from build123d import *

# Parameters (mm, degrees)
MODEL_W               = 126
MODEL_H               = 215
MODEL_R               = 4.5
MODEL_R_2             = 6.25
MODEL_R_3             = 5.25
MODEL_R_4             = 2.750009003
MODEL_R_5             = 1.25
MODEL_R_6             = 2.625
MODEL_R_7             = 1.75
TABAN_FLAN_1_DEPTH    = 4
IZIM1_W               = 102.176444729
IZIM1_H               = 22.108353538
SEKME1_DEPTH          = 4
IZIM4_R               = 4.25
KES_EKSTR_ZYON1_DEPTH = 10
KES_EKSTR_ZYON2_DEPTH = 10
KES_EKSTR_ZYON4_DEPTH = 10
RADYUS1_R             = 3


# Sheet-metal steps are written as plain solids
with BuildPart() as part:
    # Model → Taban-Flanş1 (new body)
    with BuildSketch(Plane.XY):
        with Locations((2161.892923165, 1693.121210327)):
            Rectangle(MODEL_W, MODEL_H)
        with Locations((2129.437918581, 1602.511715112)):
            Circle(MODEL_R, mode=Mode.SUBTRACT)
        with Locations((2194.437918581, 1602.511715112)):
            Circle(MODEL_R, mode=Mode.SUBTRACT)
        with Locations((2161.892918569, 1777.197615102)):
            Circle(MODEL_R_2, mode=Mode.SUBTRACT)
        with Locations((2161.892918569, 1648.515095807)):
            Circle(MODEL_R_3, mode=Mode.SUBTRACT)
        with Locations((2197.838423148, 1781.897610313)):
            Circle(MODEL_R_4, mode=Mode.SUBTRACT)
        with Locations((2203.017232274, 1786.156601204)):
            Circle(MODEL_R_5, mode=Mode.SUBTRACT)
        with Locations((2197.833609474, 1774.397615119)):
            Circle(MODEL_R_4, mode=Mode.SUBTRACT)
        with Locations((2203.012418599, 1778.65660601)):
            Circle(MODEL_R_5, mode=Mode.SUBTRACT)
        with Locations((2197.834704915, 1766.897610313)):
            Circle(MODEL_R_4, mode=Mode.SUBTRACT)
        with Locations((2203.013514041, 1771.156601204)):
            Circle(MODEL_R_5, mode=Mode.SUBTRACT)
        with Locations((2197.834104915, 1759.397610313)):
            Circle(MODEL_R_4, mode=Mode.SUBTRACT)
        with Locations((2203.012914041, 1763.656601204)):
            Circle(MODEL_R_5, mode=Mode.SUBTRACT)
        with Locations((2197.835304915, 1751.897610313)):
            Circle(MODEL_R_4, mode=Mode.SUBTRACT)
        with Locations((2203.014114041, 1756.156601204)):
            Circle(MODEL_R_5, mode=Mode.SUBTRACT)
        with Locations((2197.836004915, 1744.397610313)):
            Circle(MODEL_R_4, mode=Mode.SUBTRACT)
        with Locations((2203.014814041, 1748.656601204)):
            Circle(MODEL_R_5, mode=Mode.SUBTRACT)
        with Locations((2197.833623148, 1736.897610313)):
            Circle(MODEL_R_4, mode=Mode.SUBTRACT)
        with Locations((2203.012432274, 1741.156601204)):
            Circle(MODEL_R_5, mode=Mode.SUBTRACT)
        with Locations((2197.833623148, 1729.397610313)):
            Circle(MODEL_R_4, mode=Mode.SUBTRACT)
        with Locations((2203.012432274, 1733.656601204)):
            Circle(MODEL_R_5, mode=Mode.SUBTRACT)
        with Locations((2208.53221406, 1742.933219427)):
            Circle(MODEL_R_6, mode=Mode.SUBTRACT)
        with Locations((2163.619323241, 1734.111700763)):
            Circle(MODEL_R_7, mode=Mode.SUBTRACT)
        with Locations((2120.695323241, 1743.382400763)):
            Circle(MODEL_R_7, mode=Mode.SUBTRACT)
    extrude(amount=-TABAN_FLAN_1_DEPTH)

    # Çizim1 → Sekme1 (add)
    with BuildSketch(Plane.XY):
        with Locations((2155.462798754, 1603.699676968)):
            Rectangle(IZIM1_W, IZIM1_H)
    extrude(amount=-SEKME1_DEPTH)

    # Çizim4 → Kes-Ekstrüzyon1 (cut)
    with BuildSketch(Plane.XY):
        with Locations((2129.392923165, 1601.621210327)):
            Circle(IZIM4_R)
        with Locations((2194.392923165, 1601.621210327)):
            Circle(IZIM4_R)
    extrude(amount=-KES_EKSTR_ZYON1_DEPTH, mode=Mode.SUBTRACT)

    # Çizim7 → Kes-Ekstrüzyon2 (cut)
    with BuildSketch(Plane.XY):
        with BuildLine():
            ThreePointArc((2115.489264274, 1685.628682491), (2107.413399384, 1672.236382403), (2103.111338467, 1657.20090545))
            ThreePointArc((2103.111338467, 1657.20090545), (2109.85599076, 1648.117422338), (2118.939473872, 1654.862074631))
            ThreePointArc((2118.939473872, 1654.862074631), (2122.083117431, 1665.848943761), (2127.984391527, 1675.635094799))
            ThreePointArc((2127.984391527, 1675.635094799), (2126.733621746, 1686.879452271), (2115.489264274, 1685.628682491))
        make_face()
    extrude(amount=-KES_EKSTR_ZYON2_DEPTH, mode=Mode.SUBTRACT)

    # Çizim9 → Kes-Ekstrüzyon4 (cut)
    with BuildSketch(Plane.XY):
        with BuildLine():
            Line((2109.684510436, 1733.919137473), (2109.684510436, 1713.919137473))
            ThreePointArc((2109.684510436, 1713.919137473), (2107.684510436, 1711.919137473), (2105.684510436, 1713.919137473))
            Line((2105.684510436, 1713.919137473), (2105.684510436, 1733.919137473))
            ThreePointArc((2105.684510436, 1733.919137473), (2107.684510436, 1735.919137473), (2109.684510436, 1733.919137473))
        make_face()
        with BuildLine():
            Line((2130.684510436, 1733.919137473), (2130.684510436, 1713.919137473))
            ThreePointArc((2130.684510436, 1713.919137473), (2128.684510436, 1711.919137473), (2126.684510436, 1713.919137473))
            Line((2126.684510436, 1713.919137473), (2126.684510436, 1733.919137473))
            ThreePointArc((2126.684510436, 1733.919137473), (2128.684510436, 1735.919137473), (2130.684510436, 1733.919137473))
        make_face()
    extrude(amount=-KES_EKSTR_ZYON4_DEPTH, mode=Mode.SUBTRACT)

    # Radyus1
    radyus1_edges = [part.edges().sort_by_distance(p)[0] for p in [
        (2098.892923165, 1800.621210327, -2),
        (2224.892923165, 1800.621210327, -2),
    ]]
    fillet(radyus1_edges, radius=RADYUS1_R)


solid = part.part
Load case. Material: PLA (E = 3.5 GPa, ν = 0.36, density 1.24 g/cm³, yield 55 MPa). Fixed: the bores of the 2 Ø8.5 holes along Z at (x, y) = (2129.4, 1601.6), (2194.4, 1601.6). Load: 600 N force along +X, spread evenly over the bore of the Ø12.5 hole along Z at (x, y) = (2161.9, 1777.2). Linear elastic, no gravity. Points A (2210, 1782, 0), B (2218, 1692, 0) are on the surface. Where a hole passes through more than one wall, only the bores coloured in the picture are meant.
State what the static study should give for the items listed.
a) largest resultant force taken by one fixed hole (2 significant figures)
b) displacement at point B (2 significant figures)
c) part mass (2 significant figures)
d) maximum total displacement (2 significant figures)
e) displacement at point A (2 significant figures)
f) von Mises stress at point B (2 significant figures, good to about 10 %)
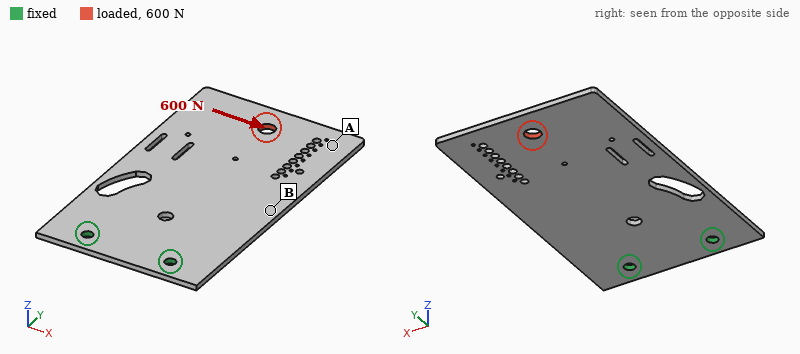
1.5 kN
0.55 mm
130 g
1.3 mm
1.2 mm
4.8 MPa
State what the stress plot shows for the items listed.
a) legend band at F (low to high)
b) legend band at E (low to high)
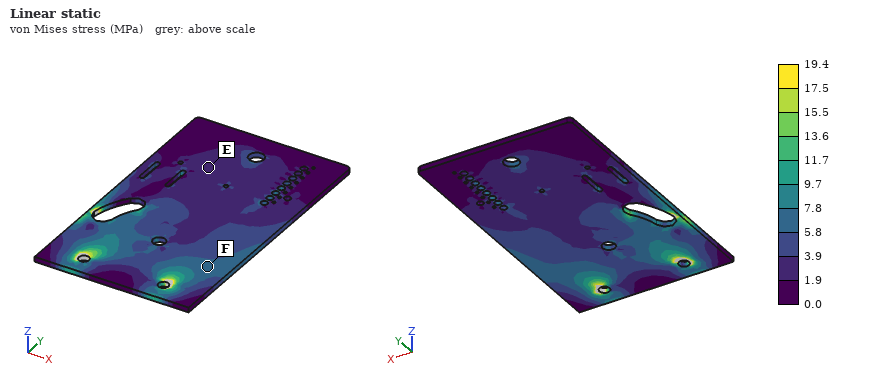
5.8 to 7.8 MPa
1.9 to 3.9 MPa
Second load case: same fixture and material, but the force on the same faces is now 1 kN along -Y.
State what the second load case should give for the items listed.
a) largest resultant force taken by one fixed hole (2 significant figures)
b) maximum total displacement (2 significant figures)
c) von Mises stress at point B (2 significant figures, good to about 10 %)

500 N
0.19 mm
1.4 MPa
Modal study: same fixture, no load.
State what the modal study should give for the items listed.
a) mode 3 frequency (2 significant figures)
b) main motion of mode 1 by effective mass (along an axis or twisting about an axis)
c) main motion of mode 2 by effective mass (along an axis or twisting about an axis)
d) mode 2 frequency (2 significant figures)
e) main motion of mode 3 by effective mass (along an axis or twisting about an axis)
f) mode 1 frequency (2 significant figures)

170 Hz
along Z
twisting about Y
93 Hz
along Z
27 Hz
